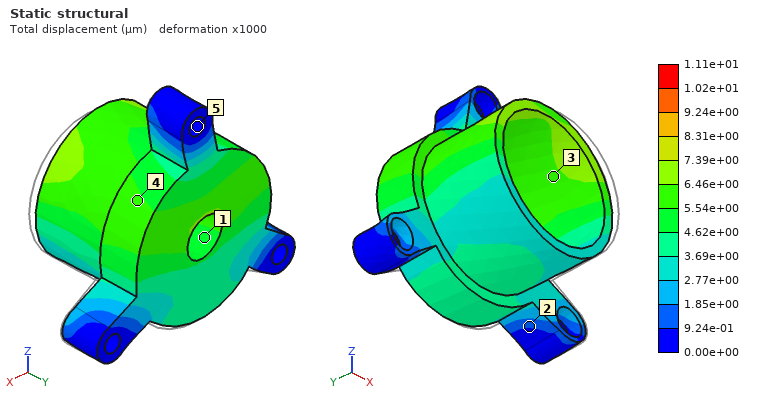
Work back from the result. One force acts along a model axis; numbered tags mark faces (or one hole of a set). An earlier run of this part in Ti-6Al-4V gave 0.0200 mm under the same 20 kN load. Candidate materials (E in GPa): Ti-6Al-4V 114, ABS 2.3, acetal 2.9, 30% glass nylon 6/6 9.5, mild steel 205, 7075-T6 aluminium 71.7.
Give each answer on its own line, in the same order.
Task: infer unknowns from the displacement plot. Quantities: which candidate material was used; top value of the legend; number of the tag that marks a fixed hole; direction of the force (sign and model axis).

mild steel
1.11e+01 µm
5
-X
